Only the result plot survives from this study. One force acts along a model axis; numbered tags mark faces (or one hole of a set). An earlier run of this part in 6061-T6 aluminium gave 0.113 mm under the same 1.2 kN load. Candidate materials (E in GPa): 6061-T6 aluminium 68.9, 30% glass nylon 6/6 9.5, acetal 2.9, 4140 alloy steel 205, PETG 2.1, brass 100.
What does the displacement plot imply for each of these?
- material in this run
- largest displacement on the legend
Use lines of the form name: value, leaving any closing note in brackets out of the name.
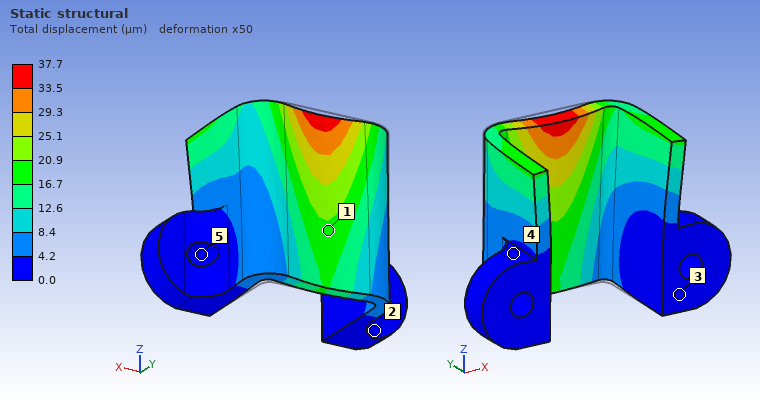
material in this run: 4140 alloy steel
largest displacement on the legend: 37.7 µm
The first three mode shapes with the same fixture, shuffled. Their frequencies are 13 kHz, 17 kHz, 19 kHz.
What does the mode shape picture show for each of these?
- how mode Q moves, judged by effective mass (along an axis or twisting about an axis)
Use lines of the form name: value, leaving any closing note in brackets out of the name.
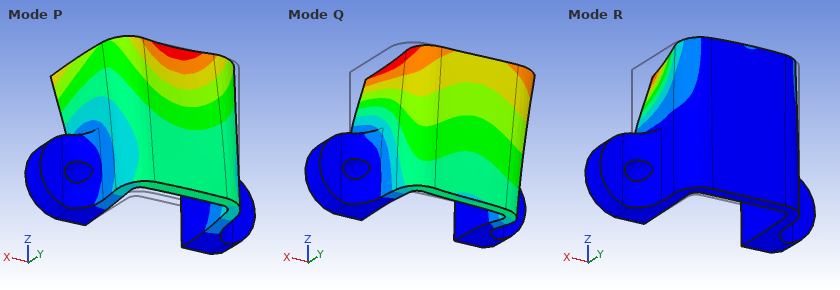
how mode Q moves, judged by effective mass: along X
